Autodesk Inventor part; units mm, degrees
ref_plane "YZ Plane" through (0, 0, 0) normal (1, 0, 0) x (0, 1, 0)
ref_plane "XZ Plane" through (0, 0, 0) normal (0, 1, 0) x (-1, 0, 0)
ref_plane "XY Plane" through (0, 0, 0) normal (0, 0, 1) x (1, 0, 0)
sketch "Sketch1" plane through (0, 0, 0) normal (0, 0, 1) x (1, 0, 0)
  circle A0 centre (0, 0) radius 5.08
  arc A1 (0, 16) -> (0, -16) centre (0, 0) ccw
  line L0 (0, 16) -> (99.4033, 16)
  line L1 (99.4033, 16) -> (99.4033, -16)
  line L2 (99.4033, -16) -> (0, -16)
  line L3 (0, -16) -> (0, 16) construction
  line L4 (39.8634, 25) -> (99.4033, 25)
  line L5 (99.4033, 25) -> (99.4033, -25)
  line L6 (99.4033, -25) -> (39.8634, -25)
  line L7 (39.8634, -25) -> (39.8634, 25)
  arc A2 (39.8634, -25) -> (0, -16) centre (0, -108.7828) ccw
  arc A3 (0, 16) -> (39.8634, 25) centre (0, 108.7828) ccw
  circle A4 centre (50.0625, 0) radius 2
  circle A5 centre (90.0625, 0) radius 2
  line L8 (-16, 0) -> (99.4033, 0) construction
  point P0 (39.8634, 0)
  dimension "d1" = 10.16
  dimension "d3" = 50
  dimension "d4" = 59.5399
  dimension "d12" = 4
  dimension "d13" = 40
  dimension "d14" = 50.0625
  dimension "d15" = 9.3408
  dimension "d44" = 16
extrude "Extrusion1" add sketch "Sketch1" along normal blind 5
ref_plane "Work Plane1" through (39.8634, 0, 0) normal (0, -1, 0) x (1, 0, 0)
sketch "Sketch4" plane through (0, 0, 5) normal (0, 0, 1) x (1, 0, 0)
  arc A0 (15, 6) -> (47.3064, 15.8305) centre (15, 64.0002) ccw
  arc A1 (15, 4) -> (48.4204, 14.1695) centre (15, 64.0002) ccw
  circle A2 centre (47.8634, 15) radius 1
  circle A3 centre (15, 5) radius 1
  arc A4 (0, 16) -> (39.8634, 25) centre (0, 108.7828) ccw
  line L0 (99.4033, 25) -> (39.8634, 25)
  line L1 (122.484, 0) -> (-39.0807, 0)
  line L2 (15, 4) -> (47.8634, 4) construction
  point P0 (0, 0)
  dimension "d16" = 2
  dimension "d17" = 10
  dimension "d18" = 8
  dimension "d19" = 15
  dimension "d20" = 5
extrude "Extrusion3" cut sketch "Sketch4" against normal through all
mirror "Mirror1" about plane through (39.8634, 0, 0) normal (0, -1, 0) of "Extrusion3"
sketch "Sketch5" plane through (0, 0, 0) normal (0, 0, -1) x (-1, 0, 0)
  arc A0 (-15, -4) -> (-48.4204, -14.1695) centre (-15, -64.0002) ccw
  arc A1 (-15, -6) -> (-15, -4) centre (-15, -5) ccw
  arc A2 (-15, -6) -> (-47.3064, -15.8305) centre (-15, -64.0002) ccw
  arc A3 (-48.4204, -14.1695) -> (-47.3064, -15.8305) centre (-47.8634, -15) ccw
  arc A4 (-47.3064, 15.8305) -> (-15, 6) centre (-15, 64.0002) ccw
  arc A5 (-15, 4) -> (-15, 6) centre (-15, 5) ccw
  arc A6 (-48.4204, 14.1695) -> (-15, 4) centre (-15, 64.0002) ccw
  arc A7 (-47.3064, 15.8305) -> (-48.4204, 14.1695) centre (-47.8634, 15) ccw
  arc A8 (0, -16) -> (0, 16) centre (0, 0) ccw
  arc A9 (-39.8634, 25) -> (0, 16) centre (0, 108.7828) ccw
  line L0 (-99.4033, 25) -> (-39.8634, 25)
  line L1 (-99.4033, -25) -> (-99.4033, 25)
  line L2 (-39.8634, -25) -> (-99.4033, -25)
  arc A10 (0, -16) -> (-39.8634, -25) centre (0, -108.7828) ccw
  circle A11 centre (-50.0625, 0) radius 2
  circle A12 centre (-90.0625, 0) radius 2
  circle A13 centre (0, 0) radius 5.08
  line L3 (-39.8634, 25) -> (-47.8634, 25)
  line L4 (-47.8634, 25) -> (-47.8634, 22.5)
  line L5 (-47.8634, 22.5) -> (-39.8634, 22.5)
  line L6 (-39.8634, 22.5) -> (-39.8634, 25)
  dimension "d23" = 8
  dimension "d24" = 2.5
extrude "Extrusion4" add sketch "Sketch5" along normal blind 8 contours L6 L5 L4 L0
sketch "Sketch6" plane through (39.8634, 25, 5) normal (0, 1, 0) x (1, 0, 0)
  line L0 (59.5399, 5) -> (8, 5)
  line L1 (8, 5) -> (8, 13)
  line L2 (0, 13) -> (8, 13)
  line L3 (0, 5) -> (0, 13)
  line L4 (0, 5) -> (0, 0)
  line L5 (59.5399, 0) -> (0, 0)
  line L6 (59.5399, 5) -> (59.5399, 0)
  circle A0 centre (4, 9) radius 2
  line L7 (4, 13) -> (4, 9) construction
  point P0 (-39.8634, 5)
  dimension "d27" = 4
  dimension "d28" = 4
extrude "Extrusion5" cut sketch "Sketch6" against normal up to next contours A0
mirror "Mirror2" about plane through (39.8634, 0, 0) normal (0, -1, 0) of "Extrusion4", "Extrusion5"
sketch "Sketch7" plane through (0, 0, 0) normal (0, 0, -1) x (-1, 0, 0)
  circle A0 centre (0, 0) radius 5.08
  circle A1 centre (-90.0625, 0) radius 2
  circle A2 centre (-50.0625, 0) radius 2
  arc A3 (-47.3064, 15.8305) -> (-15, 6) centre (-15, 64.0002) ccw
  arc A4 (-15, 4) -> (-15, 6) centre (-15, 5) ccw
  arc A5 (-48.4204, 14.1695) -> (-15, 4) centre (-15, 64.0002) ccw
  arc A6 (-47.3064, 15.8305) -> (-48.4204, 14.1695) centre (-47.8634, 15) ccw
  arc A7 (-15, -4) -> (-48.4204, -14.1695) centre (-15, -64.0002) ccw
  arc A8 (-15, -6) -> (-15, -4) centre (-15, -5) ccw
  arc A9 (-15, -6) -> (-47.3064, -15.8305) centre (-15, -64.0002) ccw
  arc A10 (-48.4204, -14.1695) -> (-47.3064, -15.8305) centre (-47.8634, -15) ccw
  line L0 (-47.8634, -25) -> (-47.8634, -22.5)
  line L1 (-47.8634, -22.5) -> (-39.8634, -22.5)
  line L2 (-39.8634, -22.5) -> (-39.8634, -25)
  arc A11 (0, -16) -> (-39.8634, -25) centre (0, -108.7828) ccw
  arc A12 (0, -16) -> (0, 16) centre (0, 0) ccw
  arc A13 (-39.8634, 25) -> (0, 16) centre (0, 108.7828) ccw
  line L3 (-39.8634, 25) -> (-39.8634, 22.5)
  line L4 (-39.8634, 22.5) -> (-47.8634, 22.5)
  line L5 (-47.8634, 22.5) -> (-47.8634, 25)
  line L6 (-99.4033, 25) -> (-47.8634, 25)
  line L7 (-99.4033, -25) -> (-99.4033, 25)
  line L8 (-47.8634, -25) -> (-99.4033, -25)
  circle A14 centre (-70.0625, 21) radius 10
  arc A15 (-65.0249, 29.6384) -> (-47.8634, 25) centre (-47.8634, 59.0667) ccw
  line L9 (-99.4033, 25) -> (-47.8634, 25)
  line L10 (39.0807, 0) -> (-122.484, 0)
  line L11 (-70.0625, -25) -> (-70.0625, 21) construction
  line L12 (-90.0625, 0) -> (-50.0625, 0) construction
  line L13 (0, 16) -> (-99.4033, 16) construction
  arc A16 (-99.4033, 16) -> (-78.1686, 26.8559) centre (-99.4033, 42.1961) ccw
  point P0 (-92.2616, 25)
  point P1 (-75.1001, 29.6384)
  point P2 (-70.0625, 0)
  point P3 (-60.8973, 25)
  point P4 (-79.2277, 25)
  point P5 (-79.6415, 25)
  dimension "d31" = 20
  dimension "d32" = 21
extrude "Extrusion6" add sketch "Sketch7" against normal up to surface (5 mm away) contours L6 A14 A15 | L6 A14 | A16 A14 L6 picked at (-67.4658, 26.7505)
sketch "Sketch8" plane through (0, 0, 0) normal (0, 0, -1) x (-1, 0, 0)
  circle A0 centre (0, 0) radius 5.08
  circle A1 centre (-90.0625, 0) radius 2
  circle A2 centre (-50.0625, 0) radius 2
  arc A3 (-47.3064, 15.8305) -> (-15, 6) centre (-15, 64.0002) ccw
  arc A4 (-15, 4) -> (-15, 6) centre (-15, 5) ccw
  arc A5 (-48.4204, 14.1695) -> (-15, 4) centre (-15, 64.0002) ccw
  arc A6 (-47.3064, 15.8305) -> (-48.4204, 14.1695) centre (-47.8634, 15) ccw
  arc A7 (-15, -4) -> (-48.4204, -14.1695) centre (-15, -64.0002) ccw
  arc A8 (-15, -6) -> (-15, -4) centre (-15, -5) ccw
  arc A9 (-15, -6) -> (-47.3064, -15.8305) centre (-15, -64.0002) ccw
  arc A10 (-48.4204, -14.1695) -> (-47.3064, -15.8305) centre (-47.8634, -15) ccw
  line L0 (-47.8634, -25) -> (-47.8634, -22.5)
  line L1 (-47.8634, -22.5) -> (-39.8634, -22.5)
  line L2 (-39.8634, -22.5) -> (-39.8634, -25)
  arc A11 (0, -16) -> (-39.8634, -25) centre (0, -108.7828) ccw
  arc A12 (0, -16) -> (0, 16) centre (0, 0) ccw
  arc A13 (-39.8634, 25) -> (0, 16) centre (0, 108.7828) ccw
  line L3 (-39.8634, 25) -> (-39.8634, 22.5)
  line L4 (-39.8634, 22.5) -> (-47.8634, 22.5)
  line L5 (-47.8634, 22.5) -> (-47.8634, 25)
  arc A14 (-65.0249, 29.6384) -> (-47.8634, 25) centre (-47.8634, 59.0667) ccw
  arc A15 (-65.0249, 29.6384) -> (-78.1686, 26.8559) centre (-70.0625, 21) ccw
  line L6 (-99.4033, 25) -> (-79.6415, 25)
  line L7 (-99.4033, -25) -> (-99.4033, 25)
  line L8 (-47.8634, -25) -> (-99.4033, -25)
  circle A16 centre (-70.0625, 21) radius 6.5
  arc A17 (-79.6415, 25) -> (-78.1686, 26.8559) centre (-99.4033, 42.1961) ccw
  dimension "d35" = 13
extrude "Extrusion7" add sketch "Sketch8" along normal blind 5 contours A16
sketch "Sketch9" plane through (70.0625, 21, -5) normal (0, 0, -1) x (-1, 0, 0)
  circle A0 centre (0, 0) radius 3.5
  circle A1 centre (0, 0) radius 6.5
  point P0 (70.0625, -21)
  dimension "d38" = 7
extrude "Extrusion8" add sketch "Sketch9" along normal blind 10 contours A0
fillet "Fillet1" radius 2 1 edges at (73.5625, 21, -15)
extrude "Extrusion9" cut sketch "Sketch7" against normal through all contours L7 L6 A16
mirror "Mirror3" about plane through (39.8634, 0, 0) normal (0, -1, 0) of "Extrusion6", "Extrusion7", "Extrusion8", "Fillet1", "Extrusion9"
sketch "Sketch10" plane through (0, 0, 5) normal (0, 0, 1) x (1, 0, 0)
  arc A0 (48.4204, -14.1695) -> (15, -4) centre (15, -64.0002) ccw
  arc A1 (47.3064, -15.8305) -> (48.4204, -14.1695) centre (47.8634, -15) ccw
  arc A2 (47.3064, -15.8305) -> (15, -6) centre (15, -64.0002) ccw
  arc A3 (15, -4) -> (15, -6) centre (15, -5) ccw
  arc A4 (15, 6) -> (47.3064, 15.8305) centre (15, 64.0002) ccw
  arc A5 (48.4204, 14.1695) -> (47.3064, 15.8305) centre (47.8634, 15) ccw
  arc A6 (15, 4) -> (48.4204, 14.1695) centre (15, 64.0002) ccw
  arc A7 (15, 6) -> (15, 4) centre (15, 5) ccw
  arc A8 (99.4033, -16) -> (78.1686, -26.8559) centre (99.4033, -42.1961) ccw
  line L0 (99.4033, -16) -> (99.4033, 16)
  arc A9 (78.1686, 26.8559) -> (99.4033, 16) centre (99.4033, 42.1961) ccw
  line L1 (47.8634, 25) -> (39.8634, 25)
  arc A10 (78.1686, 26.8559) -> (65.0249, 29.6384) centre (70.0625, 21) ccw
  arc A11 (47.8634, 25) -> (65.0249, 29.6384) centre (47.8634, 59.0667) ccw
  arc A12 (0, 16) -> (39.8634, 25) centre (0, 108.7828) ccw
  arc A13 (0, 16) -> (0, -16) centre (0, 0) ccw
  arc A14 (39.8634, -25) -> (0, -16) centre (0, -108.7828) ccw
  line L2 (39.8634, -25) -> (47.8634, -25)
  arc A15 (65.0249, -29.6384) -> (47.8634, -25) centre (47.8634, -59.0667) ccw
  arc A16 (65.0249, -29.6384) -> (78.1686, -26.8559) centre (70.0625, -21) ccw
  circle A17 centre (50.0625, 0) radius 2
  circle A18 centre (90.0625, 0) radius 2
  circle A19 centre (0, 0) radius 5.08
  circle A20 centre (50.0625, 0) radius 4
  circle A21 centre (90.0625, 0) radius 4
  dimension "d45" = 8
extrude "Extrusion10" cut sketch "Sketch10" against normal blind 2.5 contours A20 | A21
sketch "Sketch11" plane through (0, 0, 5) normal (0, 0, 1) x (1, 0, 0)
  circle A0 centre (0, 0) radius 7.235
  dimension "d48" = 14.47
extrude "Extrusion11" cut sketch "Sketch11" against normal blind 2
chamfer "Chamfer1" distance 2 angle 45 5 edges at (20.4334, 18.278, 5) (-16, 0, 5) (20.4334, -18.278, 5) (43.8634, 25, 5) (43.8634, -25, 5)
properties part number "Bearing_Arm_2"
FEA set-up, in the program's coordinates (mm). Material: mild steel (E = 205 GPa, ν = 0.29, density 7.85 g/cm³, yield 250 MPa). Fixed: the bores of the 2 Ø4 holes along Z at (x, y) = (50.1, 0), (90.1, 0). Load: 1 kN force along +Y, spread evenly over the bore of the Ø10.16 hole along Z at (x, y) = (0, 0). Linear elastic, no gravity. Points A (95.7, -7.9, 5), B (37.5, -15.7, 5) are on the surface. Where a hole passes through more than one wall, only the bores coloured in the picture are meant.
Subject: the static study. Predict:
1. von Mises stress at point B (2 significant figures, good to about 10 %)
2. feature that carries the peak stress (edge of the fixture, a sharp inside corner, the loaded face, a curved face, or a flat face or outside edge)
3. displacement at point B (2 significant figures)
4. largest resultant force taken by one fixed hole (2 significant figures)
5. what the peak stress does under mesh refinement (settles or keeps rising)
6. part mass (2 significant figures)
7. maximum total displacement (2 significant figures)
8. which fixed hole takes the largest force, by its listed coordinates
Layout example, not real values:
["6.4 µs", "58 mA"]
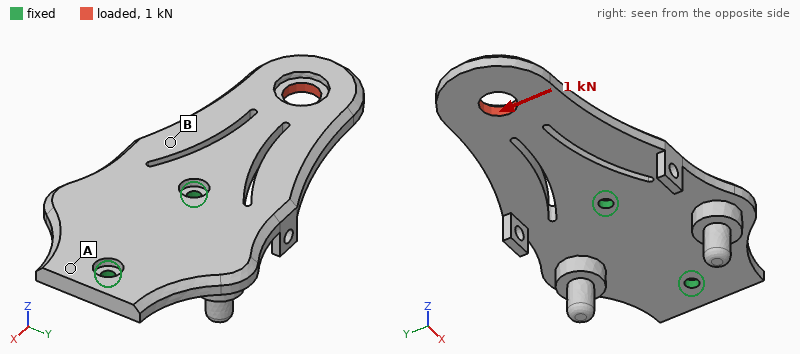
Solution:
["17 MPa", "edge of the fixture", "8.3 µm", "2.2 kN", "keeps rising", "190 g", "31 µm", "(50.1, 0)"]
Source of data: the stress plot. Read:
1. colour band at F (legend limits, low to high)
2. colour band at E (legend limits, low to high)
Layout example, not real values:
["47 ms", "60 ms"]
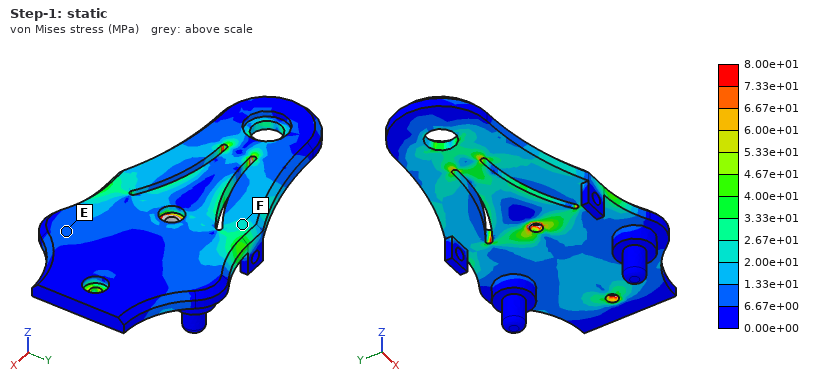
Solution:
["2.00e+01 to 2.67e+01 MPa", "6.67e+00 to 1.33e+01 MPa"]
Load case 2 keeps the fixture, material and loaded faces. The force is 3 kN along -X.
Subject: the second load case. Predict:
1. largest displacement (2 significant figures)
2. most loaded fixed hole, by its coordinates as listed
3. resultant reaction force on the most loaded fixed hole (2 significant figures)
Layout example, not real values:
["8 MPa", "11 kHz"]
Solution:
["82 µm", "(50.1, 0)", "2.1 kN"]
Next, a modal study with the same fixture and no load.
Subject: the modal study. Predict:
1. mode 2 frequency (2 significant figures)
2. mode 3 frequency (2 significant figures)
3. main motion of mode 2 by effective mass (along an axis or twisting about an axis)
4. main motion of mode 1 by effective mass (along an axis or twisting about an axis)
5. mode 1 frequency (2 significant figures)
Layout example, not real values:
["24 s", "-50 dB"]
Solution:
["2000 Hz", "3900 Hz", "twisting about X", "along Z", "1000 Hz"]
